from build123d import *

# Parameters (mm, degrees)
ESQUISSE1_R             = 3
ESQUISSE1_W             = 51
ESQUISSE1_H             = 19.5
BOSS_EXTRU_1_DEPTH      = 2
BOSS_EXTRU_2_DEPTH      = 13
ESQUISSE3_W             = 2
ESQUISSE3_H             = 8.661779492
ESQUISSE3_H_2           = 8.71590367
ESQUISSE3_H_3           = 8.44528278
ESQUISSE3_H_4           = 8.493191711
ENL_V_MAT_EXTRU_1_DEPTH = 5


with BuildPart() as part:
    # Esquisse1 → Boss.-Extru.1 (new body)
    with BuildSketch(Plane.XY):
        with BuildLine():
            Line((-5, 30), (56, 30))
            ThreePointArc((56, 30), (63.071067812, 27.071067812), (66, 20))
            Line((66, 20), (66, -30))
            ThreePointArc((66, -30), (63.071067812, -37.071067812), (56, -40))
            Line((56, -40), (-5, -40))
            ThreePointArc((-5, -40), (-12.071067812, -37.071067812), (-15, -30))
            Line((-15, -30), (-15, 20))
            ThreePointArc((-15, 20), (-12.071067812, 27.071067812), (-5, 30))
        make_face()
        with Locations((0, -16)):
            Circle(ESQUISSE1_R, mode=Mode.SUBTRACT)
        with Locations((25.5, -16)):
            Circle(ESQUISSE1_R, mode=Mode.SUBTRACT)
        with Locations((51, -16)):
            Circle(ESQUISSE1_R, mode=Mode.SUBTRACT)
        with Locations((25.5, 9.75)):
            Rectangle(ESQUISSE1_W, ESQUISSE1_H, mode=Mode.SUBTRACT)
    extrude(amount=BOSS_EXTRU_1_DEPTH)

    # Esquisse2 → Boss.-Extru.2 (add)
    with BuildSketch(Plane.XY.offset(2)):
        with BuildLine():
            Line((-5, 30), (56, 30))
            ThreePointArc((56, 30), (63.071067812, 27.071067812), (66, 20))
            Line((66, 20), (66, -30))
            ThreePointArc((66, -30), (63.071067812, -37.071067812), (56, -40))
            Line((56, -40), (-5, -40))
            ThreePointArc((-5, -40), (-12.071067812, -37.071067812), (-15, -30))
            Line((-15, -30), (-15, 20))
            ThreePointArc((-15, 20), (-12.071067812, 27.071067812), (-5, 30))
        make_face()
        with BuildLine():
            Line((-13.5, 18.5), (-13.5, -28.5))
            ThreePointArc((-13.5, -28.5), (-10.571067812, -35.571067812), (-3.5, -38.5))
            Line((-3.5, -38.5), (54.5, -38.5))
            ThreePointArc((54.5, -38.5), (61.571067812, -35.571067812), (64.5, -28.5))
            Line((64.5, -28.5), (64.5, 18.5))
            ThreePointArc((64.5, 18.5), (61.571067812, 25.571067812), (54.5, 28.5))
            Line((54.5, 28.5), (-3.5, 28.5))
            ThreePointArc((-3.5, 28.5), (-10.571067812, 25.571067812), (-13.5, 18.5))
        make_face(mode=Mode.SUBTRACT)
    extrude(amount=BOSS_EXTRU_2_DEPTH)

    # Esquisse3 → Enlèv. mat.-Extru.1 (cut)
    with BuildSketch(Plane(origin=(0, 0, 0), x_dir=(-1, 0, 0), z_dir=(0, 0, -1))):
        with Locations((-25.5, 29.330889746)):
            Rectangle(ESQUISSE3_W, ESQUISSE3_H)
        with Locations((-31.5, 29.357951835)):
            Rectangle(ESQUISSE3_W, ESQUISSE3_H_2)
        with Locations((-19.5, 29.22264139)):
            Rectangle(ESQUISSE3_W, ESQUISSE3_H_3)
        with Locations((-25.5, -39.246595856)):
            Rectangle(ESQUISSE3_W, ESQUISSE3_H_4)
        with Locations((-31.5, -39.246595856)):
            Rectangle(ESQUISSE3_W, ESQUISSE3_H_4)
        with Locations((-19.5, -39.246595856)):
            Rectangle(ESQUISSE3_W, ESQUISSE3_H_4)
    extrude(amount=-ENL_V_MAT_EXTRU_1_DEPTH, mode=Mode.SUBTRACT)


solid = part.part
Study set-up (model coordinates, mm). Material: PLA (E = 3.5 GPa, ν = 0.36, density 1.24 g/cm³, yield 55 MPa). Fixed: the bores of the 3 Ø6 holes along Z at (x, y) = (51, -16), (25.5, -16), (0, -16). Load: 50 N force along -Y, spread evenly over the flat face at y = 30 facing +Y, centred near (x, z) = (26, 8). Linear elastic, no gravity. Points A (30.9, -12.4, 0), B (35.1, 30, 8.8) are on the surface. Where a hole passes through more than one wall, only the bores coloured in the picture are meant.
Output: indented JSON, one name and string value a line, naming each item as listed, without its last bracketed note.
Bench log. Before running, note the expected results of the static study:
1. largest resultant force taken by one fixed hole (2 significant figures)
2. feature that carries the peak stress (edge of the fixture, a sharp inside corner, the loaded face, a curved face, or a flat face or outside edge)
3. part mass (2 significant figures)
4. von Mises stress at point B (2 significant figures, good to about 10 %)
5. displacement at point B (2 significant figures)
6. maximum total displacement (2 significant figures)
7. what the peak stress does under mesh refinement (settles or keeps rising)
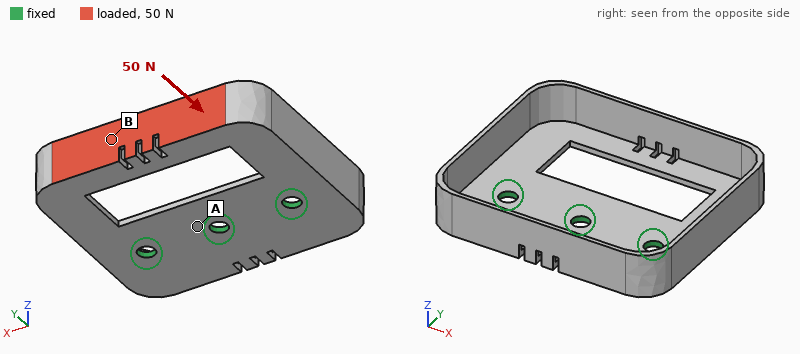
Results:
{
  "largest resultant force taken by one fixed hole": "35 N",
  "feature that carries the peak stress": "a sharp inside corner",
  "part mass": "18 g",
  "von Mises stress at point B": "5.7 MPa",
  "displacement at point B": "0.79 mm",
  "maximum total displacement": "1.2 mm",
  "what the peak stress does under mesh refinement": "keeps rising"
}
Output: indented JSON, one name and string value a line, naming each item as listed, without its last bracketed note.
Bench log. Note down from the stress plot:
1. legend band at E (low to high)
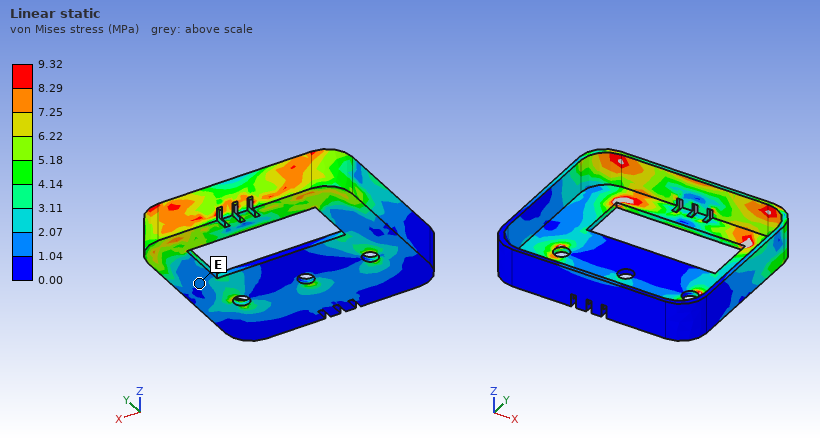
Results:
{
  "legend band at E": "1.04 to 2.07 MPa"
}
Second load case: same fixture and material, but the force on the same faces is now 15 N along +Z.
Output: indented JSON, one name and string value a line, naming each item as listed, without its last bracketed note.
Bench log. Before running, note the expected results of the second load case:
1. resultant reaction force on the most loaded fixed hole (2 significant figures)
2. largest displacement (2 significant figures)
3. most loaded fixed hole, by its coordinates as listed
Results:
{
  "resultant reaction force on the most loaded fixed hole": "16 N",
  "largest displacement": "1.0 mm",
  "most loaded fixed hole, by its coordinates as listed": "(25.5, -16)"
}
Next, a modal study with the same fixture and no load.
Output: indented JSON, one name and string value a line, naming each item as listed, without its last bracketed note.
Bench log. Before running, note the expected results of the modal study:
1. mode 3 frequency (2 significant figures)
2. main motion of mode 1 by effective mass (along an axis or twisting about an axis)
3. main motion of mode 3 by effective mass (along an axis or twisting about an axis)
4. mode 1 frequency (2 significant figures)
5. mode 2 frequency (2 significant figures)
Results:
{
  "mode 3 frequency": "990 Hz",
  "main motion of mode 1 by effective mass": "along Z",
  "main motion of mode 3 by effective mass": "along Z",
  "mode 1 frequency": "290 Hz",
  "mode 2 frequency": "360 Hz"
}
